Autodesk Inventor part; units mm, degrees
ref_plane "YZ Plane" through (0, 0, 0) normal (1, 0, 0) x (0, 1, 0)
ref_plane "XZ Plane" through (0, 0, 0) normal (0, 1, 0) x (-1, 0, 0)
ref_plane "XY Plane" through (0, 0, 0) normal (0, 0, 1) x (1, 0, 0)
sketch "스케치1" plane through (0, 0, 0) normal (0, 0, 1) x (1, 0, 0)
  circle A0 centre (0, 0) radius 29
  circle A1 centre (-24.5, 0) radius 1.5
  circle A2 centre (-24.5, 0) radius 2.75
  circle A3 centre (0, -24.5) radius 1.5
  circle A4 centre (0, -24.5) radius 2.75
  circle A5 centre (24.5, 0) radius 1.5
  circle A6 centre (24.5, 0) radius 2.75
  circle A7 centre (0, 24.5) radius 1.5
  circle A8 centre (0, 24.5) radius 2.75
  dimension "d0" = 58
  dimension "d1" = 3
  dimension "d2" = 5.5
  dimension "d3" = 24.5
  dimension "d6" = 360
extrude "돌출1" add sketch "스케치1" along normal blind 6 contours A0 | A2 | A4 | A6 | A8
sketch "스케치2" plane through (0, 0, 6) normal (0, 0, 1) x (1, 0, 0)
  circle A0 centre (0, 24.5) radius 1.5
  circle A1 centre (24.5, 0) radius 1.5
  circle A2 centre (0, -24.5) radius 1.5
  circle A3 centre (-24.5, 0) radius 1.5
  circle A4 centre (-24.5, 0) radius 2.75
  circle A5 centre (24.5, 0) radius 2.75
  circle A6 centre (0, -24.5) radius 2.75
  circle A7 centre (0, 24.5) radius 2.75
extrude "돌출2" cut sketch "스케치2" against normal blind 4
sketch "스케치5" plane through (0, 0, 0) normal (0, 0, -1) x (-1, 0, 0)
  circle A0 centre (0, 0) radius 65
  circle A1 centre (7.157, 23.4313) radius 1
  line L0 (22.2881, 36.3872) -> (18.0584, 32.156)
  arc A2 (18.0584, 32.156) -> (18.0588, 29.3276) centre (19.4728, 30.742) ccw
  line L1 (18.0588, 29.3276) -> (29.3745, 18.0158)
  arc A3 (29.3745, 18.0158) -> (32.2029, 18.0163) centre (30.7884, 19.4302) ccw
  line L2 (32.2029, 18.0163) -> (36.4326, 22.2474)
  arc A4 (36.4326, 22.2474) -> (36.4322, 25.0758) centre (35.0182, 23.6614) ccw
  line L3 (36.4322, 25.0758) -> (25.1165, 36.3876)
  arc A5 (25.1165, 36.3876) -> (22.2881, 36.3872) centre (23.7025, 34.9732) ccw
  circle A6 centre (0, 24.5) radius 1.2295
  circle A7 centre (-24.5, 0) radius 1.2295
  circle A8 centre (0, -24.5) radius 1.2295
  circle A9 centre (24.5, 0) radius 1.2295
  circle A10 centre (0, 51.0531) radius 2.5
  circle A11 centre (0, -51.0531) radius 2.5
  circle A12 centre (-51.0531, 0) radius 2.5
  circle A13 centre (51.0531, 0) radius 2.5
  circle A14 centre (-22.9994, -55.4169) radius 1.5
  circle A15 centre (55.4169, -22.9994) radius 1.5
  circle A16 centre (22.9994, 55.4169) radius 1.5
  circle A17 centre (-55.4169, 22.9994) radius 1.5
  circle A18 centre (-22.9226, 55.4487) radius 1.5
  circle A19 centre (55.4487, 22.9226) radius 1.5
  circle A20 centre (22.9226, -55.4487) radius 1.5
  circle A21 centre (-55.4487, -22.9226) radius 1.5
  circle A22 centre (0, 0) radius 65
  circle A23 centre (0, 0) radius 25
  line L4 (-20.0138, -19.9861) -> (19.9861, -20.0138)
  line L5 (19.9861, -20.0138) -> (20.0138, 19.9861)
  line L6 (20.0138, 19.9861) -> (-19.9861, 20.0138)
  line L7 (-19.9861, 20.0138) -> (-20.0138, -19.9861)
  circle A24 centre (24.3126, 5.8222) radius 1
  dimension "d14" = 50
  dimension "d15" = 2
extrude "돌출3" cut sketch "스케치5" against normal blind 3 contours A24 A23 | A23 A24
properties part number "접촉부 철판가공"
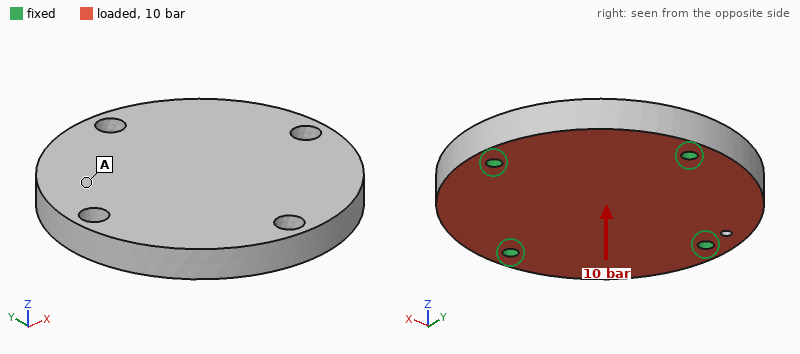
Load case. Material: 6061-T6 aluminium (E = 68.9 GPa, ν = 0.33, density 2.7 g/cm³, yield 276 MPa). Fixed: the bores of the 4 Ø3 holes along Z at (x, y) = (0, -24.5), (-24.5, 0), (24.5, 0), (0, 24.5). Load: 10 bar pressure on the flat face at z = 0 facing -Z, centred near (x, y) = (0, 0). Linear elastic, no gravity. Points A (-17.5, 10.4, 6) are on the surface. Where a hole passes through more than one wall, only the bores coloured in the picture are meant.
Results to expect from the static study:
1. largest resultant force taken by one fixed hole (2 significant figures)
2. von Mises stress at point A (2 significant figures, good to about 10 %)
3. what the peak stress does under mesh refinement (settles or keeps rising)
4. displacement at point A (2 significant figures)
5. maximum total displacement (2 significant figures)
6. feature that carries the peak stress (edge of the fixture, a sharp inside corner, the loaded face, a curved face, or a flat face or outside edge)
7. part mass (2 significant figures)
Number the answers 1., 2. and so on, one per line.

1. 740 N
2. 15 MPa
3. keeps rising
4. 9.1 µm
5. 15 µm
6. edge of the fixture
7. 42 g
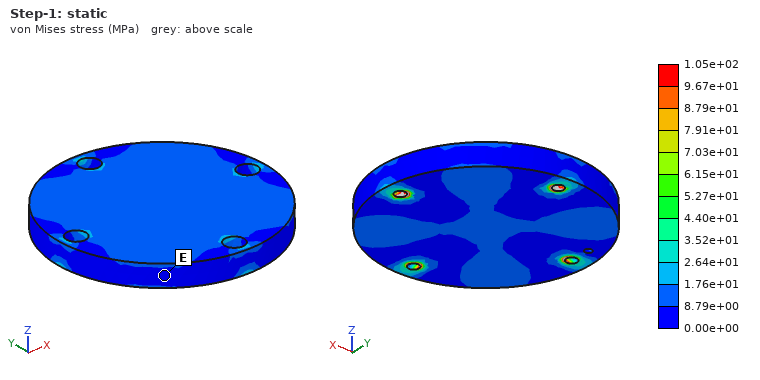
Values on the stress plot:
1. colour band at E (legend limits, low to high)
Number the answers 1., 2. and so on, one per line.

1. 0.00e+00 to 8.79e+00 MPa
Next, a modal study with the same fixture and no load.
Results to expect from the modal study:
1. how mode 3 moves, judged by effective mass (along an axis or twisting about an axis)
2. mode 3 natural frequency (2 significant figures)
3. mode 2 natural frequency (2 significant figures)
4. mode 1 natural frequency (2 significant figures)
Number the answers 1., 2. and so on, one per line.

1. twisting about Y
2. 14 kHz
3. 12 kHz
4. 12 kHz
